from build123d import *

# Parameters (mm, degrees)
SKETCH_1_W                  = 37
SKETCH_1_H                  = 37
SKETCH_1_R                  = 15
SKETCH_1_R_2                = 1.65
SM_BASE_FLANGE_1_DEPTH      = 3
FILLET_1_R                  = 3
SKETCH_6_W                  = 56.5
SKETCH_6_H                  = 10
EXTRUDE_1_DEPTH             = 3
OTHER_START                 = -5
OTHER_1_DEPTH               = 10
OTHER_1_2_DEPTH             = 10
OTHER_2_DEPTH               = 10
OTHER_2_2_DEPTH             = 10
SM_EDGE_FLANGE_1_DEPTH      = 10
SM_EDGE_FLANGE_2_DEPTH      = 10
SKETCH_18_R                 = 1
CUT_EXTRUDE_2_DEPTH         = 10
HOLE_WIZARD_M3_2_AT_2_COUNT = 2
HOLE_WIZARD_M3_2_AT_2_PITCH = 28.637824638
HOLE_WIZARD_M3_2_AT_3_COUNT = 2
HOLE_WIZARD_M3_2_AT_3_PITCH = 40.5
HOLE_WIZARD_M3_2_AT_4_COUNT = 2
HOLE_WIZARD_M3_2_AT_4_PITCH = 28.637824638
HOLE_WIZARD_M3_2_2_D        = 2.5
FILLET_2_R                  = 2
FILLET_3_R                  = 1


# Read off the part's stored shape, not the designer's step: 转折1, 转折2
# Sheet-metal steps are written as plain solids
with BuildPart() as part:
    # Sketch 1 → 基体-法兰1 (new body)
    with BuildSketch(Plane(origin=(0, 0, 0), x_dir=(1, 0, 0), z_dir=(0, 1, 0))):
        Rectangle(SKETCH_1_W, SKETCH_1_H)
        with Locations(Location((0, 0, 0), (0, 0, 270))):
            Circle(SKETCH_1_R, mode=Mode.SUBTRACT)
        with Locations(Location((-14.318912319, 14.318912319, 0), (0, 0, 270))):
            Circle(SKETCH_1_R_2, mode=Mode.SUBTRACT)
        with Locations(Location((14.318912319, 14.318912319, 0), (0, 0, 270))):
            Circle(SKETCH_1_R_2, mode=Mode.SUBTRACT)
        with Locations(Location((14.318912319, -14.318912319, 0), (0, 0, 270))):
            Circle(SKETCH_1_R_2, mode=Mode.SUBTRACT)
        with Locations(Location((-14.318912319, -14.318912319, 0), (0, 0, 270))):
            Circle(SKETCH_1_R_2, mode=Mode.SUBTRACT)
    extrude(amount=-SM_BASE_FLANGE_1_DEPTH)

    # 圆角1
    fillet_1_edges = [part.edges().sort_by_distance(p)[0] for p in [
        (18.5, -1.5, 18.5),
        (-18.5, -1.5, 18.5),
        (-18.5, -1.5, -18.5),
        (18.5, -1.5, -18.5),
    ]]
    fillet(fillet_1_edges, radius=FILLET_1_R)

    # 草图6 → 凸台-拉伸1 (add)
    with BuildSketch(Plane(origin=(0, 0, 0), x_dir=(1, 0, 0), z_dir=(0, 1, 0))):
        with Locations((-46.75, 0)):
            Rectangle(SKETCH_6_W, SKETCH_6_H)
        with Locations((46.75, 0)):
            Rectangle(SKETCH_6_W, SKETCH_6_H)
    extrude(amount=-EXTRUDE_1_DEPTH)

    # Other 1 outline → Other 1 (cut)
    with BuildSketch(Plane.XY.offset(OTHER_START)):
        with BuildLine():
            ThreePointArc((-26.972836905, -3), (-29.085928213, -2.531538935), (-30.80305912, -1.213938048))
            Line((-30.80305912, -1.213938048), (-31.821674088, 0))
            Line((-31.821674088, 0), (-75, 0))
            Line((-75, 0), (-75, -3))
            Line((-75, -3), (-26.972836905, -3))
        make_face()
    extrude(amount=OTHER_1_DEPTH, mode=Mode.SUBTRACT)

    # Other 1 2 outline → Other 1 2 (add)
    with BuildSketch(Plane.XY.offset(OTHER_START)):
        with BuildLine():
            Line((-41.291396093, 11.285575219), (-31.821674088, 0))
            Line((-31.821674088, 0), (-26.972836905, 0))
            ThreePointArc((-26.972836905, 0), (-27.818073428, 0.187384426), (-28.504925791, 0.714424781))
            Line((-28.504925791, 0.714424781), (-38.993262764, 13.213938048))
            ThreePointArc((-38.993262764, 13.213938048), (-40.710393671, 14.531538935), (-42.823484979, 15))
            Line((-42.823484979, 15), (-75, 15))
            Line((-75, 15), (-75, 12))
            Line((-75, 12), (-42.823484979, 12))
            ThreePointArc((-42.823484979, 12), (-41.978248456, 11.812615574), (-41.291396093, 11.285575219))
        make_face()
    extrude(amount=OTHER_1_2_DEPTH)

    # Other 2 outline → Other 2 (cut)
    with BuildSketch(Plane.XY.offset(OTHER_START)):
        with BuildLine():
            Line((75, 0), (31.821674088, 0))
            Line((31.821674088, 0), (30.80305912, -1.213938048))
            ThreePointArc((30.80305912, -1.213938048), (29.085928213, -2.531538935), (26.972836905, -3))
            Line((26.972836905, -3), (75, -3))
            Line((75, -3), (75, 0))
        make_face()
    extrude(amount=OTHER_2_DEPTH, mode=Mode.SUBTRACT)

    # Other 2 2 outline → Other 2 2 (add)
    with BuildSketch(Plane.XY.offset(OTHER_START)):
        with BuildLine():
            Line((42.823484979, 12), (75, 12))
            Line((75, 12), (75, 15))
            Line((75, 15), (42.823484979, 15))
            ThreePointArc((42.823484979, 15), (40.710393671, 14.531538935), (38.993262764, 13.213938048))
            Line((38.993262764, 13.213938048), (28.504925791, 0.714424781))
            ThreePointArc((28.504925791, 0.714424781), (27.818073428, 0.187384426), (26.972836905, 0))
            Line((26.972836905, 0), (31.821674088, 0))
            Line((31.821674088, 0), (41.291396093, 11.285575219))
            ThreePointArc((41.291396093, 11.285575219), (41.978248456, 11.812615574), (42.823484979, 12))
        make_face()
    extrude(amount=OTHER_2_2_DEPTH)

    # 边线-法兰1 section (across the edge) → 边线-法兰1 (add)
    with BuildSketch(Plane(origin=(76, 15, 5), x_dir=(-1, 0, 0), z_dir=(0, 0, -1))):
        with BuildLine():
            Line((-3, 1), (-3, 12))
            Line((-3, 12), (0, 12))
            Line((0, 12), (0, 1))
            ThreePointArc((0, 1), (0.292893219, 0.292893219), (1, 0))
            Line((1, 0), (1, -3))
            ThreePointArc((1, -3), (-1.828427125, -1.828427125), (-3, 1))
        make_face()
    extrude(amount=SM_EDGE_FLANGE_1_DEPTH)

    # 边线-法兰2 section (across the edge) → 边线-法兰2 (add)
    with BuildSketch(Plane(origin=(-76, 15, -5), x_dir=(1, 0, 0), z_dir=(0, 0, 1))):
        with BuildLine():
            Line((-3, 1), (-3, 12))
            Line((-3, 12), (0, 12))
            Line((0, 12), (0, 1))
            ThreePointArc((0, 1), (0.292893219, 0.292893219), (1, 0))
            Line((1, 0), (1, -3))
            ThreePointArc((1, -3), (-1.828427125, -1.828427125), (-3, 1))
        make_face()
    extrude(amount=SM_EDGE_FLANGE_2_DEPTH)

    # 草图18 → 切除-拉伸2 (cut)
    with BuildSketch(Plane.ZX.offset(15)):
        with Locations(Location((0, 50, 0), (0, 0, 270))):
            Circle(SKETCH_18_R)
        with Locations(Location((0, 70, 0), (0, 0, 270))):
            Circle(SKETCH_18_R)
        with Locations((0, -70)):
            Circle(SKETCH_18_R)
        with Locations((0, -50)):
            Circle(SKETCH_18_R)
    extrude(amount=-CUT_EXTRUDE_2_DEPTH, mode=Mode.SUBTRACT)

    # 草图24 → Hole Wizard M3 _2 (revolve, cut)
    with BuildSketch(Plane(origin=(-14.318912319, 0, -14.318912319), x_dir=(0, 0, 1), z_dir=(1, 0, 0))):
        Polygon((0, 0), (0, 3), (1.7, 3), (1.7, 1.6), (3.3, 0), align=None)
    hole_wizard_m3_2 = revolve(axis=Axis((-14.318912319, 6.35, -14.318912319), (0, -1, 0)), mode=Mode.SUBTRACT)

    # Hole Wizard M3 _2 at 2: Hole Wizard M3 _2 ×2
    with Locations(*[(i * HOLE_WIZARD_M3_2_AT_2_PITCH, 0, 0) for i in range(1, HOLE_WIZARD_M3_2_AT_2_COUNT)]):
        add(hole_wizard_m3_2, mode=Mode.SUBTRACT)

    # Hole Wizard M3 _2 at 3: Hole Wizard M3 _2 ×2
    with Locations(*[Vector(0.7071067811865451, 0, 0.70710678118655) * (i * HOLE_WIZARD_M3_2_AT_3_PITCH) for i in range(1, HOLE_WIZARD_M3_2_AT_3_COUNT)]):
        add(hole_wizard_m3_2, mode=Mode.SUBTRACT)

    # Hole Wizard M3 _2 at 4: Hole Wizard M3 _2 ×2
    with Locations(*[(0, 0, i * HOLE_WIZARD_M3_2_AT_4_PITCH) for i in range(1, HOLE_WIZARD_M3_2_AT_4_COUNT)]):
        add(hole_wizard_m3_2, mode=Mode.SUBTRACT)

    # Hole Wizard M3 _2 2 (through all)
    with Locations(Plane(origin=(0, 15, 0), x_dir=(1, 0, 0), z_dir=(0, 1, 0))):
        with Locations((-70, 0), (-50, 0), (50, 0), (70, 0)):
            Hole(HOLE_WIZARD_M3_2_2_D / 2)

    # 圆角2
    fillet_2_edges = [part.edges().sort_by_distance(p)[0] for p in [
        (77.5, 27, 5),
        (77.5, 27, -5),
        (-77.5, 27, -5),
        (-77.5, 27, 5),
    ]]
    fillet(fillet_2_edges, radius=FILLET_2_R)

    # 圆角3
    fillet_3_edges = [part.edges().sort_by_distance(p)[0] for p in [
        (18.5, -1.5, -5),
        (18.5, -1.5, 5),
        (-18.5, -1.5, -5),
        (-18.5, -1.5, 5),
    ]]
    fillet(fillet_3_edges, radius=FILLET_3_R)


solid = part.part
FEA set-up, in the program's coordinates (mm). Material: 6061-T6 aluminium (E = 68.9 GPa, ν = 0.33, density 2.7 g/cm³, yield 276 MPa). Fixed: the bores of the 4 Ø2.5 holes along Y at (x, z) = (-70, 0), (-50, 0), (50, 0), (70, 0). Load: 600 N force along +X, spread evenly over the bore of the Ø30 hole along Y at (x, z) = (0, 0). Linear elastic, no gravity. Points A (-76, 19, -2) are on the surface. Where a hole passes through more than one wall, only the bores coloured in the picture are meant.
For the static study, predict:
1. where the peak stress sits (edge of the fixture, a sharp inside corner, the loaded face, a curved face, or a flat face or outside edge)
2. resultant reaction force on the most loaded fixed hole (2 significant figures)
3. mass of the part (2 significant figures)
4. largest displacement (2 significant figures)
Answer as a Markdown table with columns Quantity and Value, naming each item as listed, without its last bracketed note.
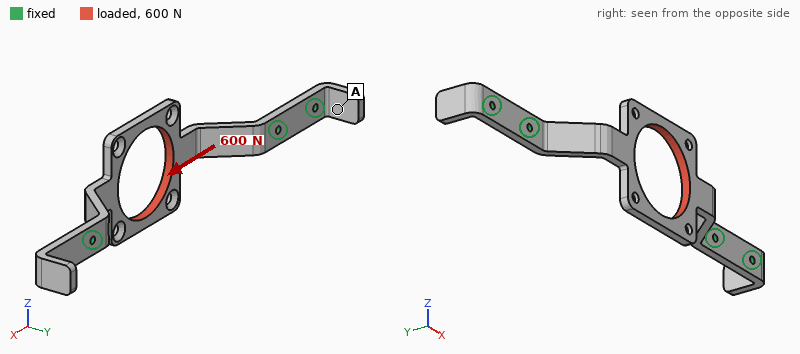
| Quantity | Value |
|---|---|
| where the peak stress sits | a curved face |
| resultant reaction force on the most loaded fixed hole | 280 N |
| mass of the part | 17 g |
| largest displacement | 0.29 mm |
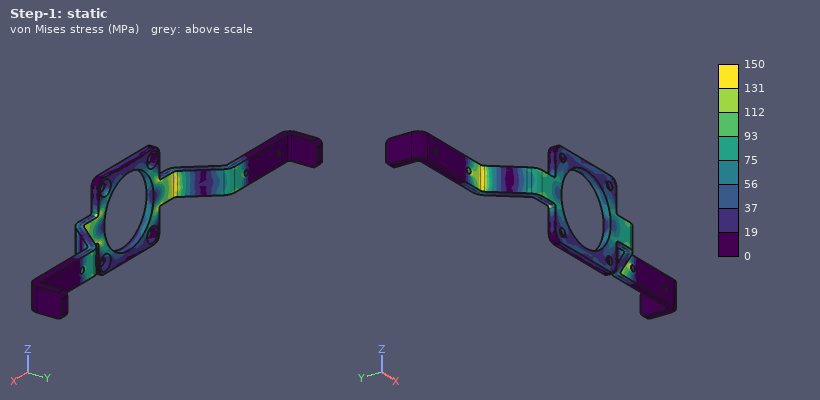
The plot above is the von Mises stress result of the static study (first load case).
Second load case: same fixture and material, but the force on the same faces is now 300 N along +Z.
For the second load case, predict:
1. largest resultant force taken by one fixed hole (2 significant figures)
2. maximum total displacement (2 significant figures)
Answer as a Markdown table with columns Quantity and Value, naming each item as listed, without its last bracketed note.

| Quantity | Value |
|---|---|
| largest resultant force taken by one fixed hole | 250 N |
| maximum total displacement | 0.30 mm |
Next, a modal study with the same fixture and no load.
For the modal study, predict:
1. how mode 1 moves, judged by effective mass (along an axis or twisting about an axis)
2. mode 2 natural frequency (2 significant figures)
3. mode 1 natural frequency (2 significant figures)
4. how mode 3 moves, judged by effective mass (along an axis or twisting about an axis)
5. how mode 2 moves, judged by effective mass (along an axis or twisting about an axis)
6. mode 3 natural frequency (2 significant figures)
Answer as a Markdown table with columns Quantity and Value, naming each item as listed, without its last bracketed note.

| Quantity | Value |
|---|---|
| how mode 1 moves, judged by effective mass | along Z |
| mode 2 natural frequency | 2200 Hz |
| mode 1 natural frequency | 1700 Hz |
| how mode 3 moves, judged by effective mass | along X |
| how mode 2 moves, judged by effective mass | along Y |
| mode 3 natural frequency | 2300 Hz |
